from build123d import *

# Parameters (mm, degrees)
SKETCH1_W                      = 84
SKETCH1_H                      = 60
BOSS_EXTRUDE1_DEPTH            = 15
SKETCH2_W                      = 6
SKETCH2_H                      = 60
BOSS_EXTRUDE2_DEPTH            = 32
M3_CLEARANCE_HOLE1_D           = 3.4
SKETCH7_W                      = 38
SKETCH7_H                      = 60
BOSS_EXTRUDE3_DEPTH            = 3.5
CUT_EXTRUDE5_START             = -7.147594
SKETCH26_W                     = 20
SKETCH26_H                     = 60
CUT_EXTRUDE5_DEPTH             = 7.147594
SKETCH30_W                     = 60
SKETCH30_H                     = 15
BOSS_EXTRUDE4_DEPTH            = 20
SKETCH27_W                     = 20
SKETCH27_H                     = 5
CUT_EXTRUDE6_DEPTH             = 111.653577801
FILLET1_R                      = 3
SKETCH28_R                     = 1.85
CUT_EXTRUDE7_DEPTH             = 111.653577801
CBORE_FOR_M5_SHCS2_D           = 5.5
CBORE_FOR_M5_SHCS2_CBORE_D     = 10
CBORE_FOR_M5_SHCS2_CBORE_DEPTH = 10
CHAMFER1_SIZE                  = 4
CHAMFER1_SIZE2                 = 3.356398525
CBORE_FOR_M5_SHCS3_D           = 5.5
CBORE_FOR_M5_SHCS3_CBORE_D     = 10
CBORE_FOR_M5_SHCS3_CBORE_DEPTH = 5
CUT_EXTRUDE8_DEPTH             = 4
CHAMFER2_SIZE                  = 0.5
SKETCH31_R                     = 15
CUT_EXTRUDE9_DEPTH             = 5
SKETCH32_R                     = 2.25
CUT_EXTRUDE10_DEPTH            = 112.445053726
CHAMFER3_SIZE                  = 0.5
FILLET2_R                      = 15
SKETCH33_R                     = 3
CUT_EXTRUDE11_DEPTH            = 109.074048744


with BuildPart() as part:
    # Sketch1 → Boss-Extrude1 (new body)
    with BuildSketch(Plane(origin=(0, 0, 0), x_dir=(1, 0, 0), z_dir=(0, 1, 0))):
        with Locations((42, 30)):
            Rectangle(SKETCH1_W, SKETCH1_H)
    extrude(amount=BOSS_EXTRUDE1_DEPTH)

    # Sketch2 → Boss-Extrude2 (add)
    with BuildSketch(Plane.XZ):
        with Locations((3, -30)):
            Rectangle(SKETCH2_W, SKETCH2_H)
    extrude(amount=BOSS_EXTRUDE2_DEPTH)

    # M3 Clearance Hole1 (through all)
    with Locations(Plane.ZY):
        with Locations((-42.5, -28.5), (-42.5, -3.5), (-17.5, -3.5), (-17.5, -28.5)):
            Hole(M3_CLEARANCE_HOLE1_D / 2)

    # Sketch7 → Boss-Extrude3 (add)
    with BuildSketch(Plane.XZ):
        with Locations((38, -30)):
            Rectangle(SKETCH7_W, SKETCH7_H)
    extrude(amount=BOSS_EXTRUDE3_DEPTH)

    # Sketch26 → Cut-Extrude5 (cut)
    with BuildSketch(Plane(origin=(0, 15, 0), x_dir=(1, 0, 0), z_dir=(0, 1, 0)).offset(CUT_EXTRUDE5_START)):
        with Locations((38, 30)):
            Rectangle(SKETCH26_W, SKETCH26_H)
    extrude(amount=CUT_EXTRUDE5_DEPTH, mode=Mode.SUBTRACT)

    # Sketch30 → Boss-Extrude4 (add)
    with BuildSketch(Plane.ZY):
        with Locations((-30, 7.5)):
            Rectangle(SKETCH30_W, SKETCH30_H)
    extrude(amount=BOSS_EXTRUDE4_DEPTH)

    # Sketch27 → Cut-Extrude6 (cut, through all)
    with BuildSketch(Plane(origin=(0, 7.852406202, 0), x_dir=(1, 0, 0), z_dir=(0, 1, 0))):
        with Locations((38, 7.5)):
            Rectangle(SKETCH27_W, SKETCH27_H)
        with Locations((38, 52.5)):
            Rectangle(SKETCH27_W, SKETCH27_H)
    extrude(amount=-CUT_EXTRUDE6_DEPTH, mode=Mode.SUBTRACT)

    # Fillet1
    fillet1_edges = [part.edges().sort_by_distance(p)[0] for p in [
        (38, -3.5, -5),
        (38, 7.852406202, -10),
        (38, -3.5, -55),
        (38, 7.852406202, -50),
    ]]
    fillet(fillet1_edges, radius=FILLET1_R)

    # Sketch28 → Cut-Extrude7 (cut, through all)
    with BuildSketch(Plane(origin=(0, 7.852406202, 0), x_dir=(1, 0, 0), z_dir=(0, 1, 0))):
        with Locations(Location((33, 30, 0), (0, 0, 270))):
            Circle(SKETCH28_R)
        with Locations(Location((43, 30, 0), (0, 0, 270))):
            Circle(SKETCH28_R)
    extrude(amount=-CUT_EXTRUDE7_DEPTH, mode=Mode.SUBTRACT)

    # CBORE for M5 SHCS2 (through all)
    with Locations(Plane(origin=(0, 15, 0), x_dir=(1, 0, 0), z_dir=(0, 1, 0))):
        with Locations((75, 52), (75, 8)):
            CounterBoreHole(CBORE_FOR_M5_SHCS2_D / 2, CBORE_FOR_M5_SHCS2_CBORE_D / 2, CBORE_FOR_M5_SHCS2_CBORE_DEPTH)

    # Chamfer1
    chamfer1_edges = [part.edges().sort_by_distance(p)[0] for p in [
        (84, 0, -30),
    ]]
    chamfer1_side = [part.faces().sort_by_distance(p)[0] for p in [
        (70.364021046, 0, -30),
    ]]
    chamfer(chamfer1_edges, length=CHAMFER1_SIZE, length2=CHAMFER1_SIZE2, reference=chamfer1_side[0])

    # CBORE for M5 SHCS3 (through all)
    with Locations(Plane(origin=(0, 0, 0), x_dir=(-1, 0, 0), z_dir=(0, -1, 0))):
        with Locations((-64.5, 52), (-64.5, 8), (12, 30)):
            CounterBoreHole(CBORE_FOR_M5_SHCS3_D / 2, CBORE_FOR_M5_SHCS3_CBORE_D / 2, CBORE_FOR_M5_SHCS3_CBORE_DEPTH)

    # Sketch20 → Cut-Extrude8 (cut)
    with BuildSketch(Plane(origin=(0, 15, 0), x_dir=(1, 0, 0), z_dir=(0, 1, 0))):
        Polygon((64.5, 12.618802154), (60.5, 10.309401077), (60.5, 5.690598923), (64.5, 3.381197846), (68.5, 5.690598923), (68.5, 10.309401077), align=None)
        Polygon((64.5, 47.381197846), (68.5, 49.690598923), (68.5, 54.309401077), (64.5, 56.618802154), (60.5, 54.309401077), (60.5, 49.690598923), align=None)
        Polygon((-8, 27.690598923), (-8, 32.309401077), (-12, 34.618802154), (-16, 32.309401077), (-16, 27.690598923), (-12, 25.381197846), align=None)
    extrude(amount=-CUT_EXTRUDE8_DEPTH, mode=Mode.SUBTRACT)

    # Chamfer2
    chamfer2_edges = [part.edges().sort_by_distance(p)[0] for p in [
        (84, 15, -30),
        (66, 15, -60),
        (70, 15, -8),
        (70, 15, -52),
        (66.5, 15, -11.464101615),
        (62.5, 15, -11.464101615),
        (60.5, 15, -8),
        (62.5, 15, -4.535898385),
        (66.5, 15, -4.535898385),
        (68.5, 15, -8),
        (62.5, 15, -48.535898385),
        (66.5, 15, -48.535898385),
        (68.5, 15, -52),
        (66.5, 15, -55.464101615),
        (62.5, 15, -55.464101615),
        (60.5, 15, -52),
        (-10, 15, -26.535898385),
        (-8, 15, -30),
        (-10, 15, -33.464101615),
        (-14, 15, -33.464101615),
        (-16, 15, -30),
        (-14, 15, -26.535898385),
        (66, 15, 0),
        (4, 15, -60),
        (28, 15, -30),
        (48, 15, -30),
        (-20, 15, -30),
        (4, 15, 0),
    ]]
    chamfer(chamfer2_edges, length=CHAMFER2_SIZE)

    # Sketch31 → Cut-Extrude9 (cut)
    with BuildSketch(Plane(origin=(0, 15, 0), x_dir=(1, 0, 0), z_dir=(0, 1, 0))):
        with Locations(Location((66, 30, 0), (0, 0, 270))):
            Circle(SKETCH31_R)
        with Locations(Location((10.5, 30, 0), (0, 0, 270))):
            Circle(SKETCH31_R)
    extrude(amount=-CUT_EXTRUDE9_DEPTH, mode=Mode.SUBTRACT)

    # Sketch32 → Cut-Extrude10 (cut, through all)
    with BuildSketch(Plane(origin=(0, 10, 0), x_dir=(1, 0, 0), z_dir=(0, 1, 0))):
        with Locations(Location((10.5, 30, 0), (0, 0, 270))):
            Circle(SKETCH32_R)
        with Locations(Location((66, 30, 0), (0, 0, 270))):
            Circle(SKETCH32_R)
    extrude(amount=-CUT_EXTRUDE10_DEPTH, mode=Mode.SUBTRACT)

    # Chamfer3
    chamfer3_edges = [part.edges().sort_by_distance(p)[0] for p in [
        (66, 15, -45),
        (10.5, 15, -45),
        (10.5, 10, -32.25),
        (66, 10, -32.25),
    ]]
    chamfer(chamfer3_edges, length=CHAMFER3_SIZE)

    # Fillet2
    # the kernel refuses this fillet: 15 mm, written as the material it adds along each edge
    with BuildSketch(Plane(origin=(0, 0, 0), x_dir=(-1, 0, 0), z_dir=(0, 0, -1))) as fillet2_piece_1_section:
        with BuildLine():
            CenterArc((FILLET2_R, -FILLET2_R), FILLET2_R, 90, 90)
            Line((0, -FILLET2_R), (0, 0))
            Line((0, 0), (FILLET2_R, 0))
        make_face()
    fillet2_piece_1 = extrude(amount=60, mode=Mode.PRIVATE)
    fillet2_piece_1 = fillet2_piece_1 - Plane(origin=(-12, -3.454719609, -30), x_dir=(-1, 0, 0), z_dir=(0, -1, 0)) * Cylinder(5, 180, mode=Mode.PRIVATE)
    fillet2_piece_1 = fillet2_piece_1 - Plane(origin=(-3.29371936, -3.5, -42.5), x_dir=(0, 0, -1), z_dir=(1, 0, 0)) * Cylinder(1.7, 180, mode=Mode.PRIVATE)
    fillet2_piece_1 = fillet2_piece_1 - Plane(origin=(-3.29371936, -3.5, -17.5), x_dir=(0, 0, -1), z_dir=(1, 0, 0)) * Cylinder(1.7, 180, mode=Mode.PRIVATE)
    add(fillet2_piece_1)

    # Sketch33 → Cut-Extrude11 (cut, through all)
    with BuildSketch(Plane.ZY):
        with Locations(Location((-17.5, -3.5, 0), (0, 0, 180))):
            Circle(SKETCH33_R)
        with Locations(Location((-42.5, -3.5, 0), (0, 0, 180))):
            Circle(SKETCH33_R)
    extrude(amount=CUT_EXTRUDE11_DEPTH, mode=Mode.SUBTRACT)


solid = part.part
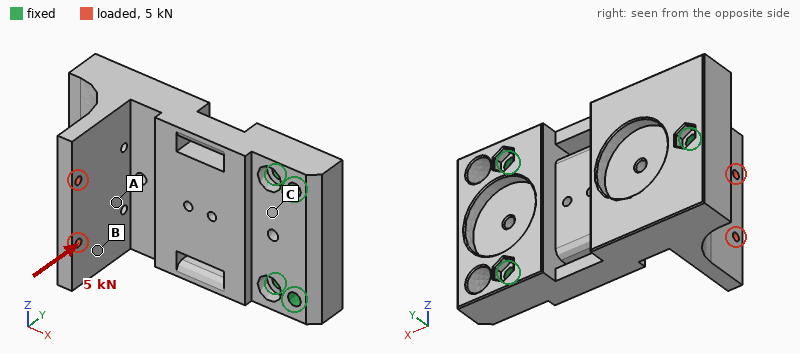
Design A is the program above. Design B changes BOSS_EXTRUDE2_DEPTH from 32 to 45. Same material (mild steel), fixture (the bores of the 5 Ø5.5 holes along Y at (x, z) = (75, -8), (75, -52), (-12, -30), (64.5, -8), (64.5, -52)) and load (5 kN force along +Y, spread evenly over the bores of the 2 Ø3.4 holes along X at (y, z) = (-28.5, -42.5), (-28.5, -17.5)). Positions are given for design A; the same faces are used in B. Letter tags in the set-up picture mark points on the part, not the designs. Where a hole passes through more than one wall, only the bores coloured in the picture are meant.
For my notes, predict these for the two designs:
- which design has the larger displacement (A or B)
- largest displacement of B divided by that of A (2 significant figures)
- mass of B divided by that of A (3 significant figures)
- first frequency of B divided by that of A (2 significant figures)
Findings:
B
1.2
1.05
0.79
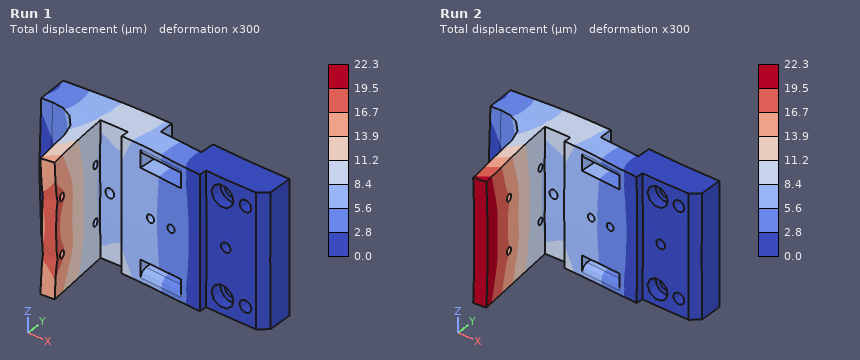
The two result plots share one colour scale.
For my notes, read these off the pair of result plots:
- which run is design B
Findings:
Run 2
